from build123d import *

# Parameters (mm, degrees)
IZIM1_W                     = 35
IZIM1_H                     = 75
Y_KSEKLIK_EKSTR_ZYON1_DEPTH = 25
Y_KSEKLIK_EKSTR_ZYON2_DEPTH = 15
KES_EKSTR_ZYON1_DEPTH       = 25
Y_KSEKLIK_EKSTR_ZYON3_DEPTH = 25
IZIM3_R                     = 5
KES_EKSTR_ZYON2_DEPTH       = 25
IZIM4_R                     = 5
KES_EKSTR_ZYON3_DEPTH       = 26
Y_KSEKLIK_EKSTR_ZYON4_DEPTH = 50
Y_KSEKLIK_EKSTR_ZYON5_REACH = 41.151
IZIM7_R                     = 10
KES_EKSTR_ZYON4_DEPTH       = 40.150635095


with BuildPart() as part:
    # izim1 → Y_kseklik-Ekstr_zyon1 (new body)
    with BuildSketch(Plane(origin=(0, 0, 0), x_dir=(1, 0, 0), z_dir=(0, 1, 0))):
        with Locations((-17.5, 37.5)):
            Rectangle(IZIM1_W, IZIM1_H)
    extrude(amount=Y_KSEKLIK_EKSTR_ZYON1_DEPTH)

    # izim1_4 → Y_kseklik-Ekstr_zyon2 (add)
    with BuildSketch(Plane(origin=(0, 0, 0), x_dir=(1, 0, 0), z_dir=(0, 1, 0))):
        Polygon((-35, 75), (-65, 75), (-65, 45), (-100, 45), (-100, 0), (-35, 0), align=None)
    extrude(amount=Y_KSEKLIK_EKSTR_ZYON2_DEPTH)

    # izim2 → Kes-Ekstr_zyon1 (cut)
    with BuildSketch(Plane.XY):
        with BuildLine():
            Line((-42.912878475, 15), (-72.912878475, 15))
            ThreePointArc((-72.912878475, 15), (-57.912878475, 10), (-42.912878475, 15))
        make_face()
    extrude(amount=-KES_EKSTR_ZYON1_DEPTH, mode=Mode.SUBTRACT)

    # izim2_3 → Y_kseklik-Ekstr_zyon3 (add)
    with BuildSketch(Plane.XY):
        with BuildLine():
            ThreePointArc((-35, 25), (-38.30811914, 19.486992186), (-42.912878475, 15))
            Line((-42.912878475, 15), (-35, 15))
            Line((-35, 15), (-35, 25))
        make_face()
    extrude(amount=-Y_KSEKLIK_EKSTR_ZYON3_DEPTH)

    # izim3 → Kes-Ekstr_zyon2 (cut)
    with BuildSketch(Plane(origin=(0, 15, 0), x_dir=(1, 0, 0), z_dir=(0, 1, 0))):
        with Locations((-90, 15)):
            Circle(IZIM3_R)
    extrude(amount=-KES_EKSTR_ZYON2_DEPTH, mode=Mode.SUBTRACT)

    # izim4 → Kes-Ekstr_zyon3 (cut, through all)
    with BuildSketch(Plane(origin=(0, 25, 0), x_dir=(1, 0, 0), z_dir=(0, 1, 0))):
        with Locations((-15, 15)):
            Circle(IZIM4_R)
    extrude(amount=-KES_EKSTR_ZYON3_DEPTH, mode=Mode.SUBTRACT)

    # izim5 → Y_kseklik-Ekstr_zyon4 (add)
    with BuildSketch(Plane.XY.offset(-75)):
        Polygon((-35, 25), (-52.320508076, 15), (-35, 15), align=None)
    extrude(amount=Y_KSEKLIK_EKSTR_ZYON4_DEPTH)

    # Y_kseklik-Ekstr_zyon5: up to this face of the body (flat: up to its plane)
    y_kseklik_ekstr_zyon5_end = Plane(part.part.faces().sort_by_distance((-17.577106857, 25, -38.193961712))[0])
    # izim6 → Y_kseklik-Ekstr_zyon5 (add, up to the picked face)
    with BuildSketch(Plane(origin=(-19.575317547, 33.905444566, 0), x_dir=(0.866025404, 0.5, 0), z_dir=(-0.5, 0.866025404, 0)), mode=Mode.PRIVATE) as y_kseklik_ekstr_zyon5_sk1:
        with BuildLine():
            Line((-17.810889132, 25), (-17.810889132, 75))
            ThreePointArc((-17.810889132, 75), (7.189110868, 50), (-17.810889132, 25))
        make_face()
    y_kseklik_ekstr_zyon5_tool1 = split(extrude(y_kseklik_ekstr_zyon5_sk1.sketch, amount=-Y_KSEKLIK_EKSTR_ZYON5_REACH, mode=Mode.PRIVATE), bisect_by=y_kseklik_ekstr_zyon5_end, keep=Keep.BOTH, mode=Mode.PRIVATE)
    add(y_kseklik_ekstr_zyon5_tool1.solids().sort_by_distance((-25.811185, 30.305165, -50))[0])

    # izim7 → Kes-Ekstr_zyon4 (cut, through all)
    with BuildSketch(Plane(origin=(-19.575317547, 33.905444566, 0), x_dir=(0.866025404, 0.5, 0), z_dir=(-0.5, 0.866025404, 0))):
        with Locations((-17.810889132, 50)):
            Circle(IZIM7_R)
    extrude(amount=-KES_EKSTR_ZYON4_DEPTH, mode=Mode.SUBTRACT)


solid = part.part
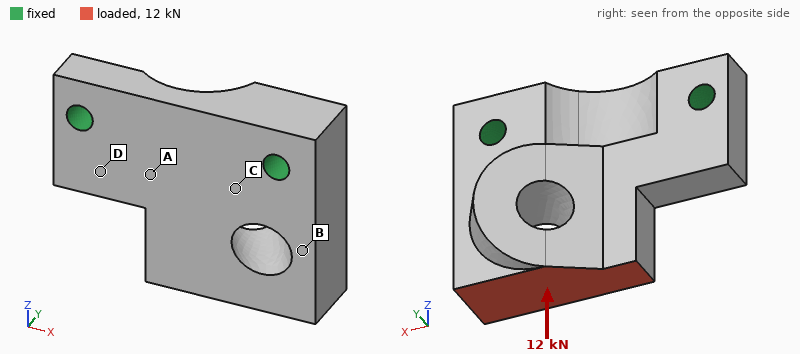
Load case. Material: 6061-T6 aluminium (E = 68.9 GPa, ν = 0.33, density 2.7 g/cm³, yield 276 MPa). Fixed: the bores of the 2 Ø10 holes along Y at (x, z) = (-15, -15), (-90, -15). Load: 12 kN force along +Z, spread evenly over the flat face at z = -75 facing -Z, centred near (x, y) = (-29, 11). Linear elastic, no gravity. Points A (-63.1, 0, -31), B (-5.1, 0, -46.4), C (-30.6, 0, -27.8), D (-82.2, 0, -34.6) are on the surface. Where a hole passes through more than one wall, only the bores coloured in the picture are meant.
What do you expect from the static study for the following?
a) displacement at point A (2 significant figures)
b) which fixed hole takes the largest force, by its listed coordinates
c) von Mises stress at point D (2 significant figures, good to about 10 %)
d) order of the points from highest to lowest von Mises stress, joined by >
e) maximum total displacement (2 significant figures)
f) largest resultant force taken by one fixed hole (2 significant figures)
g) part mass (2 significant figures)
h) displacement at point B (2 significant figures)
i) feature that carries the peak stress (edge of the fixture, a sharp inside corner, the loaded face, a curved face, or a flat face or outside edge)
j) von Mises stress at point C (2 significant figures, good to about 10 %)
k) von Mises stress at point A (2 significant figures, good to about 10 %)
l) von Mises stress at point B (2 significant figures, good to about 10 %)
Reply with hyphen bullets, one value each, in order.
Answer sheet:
- 6.6 µm
- (-15, -15)
- 5.8 MPa
- B > C > A > D
- 16 µm
- 9.8 kN
- 320 g
- 7.0 µm
- a curved face
- 14 MPa
- 8.9 MPa
- 18 MPa
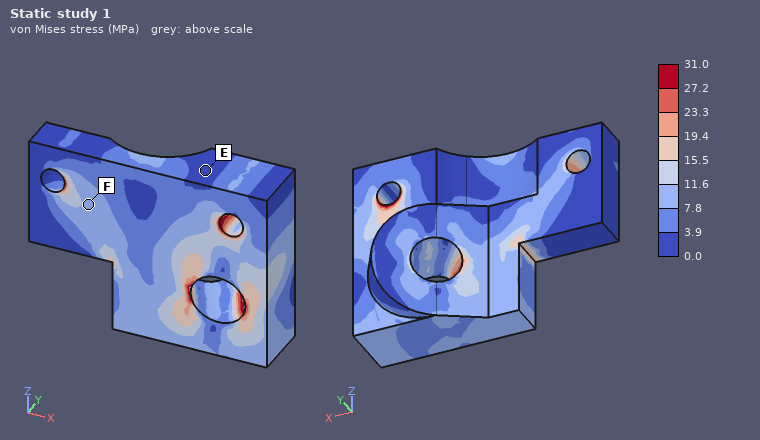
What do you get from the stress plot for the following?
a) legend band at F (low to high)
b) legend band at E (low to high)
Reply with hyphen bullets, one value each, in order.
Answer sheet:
- 7.8 to 11.6 MPa
- 0.0 to 3.9 MPa
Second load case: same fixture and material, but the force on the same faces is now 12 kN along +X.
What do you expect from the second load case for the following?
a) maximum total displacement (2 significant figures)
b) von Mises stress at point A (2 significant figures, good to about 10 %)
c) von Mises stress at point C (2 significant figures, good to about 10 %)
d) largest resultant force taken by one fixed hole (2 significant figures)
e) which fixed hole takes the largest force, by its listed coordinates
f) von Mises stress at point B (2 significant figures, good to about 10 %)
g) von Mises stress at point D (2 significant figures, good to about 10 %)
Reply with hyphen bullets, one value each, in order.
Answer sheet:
- 78 µm
- 22 MPa
- 18 MPa
- 11 kN
- (-90, -15)
- 33 MPa
- 21 MPa
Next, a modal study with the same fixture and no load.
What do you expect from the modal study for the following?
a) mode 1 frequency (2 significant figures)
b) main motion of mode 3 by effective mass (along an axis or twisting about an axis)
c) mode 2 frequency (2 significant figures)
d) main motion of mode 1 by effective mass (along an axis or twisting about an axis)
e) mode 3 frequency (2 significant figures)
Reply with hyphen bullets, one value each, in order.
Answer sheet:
- 4100 Hz
- along X
- 7700 Hz
- along Y
- 8500 Hz
